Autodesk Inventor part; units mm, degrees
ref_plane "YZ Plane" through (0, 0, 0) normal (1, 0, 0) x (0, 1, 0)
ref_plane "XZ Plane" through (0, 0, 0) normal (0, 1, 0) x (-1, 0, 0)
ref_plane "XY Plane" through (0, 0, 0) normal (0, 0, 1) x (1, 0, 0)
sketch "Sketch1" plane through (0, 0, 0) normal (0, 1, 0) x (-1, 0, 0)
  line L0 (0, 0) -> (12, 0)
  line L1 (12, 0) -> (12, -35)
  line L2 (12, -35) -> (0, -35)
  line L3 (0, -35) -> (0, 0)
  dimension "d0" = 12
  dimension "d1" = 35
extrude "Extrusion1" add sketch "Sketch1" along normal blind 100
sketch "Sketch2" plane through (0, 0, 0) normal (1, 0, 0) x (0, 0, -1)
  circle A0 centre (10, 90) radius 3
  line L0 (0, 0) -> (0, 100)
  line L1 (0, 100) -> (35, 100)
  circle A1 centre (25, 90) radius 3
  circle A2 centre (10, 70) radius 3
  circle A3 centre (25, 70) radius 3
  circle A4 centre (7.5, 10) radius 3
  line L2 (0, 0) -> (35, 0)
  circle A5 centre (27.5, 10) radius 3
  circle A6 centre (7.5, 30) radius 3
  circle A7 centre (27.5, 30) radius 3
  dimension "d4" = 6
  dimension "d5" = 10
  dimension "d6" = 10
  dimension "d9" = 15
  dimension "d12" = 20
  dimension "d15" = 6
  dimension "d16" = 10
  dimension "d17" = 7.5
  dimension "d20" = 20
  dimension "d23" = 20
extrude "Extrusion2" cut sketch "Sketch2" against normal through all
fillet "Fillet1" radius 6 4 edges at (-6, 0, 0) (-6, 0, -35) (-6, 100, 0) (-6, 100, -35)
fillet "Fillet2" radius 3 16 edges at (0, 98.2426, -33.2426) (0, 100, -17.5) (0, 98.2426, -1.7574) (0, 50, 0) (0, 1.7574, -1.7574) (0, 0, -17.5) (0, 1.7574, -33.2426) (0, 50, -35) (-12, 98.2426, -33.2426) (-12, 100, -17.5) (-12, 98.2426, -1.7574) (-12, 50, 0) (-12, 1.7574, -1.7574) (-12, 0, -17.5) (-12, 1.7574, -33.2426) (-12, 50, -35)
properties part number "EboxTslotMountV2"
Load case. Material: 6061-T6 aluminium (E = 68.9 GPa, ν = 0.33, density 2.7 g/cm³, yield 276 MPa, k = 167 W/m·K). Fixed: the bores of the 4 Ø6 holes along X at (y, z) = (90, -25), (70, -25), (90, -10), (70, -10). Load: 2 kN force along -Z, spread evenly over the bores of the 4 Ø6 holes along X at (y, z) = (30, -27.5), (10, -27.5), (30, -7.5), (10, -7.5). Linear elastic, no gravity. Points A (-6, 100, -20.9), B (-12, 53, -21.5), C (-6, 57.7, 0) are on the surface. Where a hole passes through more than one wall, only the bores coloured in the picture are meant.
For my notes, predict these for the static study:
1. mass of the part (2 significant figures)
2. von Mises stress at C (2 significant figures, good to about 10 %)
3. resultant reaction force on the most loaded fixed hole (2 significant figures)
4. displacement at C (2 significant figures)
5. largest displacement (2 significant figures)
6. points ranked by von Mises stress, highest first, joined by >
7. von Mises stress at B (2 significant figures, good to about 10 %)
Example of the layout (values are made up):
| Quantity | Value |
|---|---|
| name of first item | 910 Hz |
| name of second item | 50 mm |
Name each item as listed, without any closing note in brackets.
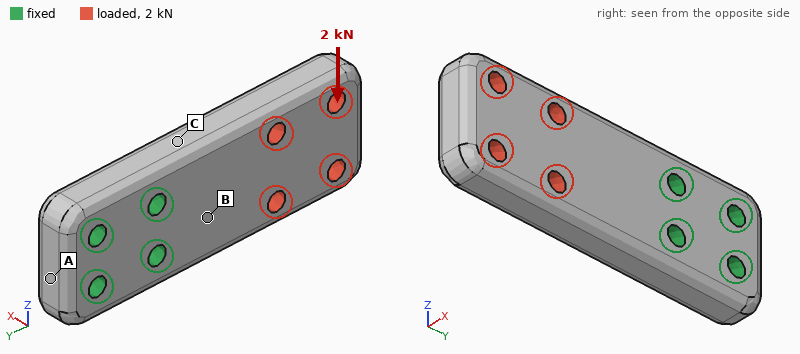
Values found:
| Quantity | Value |
|---|---|
| mass of the part | 100 g |
| von Mises stress at C | 29 MPa |
| resultant reaction force on the most loaded fixed hole | 4.2 kN |
| displacement at C | 12 µm |
| largest displacement | 70 µm |
| points ranked by von Mises stress, highest first, joined by > | C > B > A |
| von Mises stress at B | 15 MPa |
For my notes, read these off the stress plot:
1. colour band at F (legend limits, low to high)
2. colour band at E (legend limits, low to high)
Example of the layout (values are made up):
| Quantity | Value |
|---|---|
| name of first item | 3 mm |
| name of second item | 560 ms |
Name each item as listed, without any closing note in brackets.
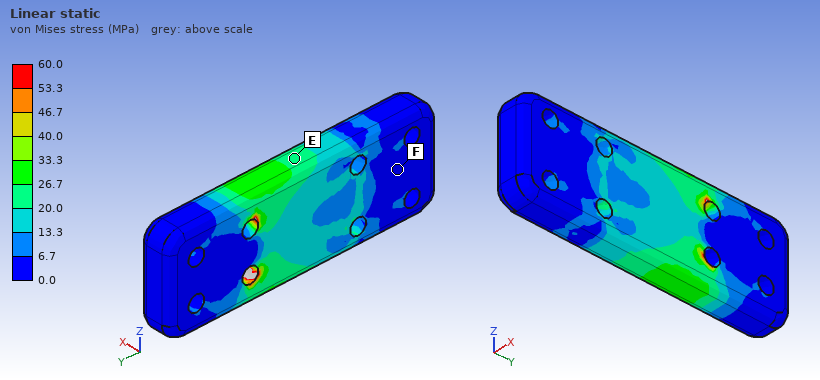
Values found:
| Quantity | Value |
|---|---|
| colour band at F | 0.0 to 6.7 MPa |
| colour band at E | 20.0 to 26.7 MPa |
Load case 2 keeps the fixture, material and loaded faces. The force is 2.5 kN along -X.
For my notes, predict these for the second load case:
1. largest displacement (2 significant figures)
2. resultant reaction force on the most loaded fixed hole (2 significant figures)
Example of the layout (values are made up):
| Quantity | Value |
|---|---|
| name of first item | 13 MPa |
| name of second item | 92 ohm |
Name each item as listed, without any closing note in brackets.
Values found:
| Quantity | Value |
|---|---|
| largest displacement | 0.50 mm |
| resultant reaction force on the most loaded fixed hole | 1.7 kN |
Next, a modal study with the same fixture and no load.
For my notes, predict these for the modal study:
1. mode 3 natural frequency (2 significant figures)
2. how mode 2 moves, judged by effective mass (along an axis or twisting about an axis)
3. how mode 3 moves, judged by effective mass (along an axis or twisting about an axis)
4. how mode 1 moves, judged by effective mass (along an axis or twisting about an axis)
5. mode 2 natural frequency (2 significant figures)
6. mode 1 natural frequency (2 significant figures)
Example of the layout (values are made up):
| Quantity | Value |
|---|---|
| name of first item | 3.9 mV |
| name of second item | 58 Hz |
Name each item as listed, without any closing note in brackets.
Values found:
| Quantity | Value |
|---|---|
| mode 3 natural frequency | 7300 Hz |
| how mode 2 moves, judged by effective mass | along Z |
| how mode 3 moves, judged by effective mass | twisting about Y |
| how mode 1 moves, judged by effective mass | along X |
| mode 2 natural frequency | 4800 Hz |
| mode 1 natural frequency | 2100 Hz |
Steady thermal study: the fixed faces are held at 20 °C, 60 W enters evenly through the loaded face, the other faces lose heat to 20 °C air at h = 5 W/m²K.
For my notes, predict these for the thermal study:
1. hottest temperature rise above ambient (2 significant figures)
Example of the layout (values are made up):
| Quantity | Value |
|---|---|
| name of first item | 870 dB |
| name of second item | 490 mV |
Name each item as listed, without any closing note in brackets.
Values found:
| Quantity | Value |
|---|---|
| hottest temperature rise above ambient | 46 K |
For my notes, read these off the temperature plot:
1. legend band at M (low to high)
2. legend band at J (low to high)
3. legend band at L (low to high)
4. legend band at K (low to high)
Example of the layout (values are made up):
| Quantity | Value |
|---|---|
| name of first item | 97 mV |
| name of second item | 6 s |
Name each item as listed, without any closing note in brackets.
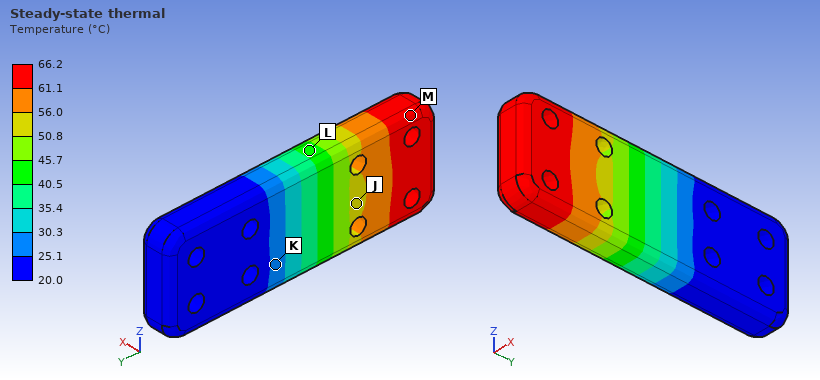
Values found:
| Quantity | Value |
|---|---|
| legend band at M | 61.1 to 66.2 °C |
| legend band at J | 50.8 to 56.0 °C |
| legend band at L | 40.5 to 45.7 °C |
| legend band at K | 25.1 to 30.3 °C |
